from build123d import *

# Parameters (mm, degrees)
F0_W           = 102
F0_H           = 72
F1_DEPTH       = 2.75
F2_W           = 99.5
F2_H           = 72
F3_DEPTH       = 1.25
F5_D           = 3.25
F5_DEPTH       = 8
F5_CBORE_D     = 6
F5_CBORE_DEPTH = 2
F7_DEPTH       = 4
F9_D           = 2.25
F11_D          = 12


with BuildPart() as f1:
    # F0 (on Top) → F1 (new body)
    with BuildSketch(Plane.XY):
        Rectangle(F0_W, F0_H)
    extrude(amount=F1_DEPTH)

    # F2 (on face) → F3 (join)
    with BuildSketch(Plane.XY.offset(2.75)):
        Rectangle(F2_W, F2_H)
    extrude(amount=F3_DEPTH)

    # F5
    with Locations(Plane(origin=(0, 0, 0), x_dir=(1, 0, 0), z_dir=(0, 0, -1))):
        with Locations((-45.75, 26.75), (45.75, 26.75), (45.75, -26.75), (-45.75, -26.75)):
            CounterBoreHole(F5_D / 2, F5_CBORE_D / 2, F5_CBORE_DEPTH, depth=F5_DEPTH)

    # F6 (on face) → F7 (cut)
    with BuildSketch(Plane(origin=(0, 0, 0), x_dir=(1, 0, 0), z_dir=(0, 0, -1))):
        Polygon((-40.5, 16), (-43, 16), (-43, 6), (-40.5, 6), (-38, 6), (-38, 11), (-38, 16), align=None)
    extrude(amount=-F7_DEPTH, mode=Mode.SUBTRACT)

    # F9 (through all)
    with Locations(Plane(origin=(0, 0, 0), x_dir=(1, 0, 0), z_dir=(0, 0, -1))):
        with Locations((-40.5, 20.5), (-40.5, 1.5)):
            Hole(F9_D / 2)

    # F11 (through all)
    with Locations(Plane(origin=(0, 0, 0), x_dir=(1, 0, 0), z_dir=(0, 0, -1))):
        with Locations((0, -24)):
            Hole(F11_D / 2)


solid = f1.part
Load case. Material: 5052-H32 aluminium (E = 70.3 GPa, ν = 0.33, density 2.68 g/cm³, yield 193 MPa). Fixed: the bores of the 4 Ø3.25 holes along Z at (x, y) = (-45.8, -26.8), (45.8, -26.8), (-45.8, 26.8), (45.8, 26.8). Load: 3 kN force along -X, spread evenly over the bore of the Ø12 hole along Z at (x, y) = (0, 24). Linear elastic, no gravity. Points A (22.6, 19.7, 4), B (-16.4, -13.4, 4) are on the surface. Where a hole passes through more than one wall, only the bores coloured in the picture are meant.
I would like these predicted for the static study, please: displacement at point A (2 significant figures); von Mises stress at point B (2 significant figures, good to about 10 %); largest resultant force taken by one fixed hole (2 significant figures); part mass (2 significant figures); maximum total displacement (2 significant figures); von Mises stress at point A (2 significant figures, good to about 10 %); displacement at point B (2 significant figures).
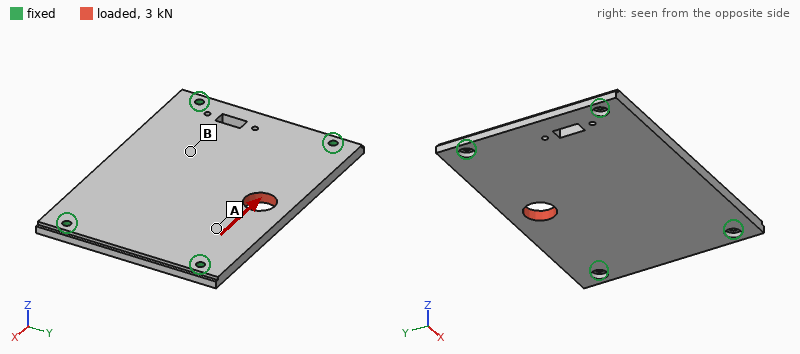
9.2 µm
4.1 MPa
1.1 kN
76 g
14 µm
14 MPa
4.6 µm
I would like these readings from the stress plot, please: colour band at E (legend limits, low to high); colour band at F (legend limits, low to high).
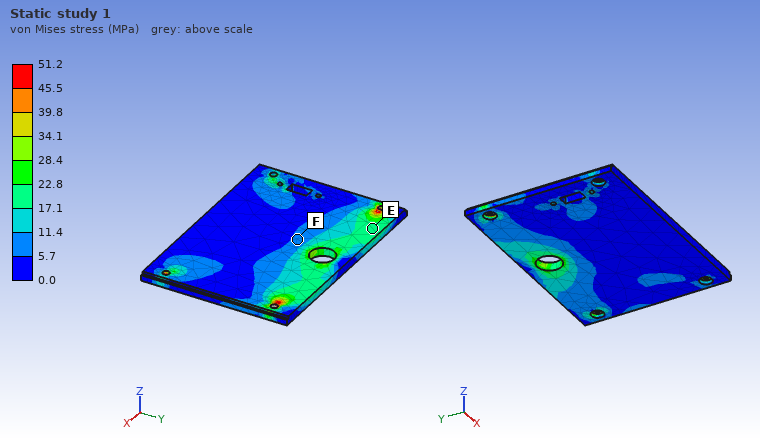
17.1 to 22.8 MPa
5.7 to 11.4 MPa
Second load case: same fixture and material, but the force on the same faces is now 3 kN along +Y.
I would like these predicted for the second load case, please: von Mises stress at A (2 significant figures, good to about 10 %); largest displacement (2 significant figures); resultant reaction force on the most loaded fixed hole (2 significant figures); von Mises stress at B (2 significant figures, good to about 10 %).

13 MPa
26 µm
930 N
11 MPa
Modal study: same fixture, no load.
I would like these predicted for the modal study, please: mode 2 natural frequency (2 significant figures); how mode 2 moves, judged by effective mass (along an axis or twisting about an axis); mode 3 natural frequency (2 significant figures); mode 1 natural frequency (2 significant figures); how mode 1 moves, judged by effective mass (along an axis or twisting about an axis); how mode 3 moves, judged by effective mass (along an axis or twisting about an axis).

2800 Hz
twisting about X
4700 Hz
1700 Hz
along Z
twisting about Y
